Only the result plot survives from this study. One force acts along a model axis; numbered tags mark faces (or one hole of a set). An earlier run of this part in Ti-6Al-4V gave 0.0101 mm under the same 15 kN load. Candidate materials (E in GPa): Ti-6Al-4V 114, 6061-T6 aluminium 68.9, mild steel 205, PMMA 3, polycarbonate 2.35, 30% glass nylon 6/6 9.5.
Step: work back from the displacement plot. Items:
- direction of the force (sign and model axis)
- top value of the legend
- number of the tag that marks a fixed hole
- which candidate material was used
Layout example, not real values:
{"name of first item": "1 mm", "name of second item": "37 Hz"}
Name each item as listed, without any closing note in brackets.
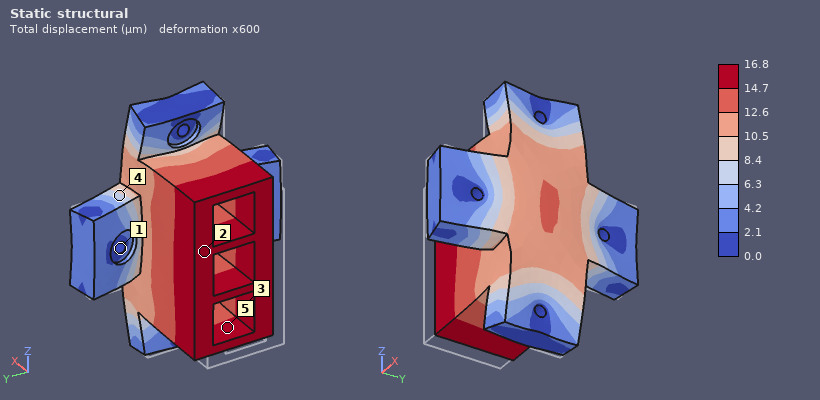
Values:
{"direction of the force": "+X", "top value of the legend": "16.8 µm", "number of the tag that marks a fixed hole": "1", "which candidate material was used": "6061-T6 aluminium"}
